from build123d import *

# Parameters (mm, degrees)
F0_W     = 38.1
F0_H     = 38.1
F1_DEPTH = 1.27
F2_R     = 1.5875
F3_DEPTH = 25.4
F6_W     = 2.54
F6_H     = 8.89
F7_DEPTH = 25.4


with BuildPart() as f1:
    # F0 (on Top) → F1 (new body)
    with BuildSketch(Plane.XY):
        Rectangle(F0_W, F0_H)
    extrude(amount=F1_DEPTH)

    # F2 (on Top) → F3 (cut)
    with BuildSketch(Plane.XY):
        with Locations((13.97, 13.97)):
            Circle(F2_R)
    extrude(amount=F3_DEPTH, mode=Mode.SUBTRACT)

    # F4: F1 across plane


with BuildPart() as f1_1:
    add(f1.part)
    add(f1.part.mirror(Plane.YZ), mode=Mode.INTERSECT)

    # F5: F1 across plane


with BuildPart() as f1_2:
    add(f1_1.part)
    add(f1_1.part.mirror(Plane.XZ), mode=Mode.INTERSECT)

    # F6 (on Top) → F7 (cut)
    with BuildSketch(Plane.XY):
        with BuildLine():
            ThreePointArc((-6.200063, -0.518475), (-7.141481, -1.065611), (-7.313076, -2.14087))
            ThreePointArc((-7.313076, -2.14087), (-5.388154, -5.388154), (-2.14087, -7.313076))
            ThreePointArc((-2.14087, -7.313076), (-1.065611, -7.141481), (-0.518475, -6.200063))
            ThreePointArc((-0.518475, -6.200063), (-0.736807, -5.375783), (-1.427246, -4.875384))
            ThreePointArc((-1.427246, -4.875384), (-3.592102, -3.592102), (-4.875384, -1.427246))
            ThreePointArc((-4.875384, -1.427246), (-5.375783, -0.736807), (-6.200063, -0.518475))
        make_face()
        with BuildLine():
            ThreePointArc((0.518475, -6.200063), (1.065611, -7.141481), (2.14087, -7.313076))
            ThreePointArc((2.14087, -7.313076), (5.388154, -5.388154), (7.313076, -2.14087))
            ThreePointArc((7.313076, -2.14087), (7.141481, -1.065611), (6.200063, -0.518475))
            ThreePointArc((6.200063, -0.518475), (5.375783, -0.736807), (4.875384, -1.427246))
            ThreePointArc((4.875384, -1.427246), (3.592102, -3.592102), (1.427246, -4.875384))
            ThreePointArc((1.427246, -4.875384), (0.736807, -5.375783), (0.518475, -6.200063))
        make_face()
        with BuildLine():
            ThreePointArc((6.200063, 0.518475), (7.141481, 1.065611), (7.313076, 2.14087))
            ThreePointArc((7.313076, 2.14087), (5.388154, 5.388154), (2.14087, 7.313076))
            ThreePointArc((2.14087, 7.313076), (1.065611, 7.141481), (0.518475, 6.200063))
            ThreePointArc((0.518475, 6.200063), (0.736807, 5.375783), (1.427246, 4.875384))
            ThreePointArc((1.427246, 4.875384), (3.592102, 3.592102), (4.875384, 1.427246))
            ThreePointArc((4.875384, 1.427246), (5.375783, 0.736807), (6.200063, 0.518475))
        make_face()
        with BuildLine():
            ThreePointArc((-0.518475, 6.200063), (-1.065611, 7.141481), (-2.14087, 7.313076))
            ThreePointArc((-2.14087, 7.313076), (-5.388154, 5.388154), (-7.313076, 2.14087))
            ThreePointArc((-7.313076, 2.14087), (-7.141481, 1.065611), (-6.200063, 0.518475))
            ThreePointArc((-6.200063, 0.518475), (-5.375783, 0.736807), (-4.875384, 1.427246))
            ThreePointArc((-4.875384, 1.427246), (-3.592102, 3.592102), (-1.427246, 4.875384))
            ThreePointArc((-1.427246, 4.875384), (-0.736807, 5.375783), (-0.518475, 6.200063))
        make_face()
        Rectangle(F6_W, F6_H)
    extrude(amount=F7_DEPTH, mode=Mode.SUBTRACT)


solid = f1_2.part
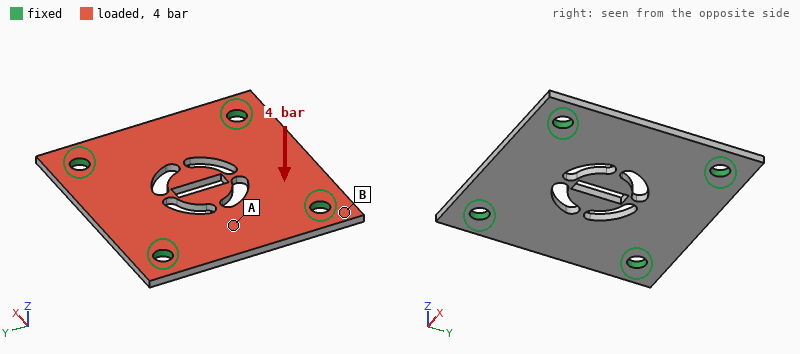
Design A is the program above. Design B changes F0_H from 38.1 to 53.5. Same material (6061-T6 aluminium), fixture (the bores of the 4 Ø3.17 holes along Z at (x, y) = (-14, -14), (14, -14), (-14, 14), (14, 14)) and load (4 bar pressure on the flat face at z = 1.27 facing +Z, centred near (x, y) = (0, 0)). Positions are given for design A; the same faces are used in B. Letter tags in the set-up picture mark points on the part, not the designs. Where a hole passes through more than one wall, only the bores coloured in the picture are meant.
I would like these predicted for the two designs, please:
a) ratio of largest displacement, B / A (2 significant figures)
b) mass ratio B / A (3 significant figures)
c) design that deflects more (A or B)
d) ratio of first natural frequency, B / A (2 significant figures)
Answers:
1.4
1.45
B
0.80
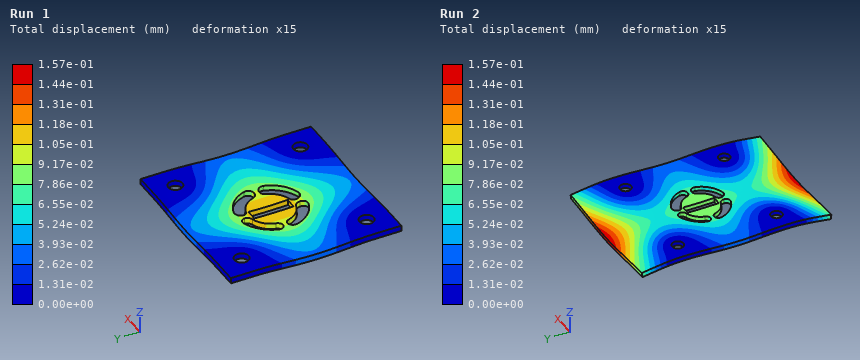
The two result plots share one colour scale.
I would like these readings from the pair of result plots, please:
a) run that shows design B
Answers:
Run 2
